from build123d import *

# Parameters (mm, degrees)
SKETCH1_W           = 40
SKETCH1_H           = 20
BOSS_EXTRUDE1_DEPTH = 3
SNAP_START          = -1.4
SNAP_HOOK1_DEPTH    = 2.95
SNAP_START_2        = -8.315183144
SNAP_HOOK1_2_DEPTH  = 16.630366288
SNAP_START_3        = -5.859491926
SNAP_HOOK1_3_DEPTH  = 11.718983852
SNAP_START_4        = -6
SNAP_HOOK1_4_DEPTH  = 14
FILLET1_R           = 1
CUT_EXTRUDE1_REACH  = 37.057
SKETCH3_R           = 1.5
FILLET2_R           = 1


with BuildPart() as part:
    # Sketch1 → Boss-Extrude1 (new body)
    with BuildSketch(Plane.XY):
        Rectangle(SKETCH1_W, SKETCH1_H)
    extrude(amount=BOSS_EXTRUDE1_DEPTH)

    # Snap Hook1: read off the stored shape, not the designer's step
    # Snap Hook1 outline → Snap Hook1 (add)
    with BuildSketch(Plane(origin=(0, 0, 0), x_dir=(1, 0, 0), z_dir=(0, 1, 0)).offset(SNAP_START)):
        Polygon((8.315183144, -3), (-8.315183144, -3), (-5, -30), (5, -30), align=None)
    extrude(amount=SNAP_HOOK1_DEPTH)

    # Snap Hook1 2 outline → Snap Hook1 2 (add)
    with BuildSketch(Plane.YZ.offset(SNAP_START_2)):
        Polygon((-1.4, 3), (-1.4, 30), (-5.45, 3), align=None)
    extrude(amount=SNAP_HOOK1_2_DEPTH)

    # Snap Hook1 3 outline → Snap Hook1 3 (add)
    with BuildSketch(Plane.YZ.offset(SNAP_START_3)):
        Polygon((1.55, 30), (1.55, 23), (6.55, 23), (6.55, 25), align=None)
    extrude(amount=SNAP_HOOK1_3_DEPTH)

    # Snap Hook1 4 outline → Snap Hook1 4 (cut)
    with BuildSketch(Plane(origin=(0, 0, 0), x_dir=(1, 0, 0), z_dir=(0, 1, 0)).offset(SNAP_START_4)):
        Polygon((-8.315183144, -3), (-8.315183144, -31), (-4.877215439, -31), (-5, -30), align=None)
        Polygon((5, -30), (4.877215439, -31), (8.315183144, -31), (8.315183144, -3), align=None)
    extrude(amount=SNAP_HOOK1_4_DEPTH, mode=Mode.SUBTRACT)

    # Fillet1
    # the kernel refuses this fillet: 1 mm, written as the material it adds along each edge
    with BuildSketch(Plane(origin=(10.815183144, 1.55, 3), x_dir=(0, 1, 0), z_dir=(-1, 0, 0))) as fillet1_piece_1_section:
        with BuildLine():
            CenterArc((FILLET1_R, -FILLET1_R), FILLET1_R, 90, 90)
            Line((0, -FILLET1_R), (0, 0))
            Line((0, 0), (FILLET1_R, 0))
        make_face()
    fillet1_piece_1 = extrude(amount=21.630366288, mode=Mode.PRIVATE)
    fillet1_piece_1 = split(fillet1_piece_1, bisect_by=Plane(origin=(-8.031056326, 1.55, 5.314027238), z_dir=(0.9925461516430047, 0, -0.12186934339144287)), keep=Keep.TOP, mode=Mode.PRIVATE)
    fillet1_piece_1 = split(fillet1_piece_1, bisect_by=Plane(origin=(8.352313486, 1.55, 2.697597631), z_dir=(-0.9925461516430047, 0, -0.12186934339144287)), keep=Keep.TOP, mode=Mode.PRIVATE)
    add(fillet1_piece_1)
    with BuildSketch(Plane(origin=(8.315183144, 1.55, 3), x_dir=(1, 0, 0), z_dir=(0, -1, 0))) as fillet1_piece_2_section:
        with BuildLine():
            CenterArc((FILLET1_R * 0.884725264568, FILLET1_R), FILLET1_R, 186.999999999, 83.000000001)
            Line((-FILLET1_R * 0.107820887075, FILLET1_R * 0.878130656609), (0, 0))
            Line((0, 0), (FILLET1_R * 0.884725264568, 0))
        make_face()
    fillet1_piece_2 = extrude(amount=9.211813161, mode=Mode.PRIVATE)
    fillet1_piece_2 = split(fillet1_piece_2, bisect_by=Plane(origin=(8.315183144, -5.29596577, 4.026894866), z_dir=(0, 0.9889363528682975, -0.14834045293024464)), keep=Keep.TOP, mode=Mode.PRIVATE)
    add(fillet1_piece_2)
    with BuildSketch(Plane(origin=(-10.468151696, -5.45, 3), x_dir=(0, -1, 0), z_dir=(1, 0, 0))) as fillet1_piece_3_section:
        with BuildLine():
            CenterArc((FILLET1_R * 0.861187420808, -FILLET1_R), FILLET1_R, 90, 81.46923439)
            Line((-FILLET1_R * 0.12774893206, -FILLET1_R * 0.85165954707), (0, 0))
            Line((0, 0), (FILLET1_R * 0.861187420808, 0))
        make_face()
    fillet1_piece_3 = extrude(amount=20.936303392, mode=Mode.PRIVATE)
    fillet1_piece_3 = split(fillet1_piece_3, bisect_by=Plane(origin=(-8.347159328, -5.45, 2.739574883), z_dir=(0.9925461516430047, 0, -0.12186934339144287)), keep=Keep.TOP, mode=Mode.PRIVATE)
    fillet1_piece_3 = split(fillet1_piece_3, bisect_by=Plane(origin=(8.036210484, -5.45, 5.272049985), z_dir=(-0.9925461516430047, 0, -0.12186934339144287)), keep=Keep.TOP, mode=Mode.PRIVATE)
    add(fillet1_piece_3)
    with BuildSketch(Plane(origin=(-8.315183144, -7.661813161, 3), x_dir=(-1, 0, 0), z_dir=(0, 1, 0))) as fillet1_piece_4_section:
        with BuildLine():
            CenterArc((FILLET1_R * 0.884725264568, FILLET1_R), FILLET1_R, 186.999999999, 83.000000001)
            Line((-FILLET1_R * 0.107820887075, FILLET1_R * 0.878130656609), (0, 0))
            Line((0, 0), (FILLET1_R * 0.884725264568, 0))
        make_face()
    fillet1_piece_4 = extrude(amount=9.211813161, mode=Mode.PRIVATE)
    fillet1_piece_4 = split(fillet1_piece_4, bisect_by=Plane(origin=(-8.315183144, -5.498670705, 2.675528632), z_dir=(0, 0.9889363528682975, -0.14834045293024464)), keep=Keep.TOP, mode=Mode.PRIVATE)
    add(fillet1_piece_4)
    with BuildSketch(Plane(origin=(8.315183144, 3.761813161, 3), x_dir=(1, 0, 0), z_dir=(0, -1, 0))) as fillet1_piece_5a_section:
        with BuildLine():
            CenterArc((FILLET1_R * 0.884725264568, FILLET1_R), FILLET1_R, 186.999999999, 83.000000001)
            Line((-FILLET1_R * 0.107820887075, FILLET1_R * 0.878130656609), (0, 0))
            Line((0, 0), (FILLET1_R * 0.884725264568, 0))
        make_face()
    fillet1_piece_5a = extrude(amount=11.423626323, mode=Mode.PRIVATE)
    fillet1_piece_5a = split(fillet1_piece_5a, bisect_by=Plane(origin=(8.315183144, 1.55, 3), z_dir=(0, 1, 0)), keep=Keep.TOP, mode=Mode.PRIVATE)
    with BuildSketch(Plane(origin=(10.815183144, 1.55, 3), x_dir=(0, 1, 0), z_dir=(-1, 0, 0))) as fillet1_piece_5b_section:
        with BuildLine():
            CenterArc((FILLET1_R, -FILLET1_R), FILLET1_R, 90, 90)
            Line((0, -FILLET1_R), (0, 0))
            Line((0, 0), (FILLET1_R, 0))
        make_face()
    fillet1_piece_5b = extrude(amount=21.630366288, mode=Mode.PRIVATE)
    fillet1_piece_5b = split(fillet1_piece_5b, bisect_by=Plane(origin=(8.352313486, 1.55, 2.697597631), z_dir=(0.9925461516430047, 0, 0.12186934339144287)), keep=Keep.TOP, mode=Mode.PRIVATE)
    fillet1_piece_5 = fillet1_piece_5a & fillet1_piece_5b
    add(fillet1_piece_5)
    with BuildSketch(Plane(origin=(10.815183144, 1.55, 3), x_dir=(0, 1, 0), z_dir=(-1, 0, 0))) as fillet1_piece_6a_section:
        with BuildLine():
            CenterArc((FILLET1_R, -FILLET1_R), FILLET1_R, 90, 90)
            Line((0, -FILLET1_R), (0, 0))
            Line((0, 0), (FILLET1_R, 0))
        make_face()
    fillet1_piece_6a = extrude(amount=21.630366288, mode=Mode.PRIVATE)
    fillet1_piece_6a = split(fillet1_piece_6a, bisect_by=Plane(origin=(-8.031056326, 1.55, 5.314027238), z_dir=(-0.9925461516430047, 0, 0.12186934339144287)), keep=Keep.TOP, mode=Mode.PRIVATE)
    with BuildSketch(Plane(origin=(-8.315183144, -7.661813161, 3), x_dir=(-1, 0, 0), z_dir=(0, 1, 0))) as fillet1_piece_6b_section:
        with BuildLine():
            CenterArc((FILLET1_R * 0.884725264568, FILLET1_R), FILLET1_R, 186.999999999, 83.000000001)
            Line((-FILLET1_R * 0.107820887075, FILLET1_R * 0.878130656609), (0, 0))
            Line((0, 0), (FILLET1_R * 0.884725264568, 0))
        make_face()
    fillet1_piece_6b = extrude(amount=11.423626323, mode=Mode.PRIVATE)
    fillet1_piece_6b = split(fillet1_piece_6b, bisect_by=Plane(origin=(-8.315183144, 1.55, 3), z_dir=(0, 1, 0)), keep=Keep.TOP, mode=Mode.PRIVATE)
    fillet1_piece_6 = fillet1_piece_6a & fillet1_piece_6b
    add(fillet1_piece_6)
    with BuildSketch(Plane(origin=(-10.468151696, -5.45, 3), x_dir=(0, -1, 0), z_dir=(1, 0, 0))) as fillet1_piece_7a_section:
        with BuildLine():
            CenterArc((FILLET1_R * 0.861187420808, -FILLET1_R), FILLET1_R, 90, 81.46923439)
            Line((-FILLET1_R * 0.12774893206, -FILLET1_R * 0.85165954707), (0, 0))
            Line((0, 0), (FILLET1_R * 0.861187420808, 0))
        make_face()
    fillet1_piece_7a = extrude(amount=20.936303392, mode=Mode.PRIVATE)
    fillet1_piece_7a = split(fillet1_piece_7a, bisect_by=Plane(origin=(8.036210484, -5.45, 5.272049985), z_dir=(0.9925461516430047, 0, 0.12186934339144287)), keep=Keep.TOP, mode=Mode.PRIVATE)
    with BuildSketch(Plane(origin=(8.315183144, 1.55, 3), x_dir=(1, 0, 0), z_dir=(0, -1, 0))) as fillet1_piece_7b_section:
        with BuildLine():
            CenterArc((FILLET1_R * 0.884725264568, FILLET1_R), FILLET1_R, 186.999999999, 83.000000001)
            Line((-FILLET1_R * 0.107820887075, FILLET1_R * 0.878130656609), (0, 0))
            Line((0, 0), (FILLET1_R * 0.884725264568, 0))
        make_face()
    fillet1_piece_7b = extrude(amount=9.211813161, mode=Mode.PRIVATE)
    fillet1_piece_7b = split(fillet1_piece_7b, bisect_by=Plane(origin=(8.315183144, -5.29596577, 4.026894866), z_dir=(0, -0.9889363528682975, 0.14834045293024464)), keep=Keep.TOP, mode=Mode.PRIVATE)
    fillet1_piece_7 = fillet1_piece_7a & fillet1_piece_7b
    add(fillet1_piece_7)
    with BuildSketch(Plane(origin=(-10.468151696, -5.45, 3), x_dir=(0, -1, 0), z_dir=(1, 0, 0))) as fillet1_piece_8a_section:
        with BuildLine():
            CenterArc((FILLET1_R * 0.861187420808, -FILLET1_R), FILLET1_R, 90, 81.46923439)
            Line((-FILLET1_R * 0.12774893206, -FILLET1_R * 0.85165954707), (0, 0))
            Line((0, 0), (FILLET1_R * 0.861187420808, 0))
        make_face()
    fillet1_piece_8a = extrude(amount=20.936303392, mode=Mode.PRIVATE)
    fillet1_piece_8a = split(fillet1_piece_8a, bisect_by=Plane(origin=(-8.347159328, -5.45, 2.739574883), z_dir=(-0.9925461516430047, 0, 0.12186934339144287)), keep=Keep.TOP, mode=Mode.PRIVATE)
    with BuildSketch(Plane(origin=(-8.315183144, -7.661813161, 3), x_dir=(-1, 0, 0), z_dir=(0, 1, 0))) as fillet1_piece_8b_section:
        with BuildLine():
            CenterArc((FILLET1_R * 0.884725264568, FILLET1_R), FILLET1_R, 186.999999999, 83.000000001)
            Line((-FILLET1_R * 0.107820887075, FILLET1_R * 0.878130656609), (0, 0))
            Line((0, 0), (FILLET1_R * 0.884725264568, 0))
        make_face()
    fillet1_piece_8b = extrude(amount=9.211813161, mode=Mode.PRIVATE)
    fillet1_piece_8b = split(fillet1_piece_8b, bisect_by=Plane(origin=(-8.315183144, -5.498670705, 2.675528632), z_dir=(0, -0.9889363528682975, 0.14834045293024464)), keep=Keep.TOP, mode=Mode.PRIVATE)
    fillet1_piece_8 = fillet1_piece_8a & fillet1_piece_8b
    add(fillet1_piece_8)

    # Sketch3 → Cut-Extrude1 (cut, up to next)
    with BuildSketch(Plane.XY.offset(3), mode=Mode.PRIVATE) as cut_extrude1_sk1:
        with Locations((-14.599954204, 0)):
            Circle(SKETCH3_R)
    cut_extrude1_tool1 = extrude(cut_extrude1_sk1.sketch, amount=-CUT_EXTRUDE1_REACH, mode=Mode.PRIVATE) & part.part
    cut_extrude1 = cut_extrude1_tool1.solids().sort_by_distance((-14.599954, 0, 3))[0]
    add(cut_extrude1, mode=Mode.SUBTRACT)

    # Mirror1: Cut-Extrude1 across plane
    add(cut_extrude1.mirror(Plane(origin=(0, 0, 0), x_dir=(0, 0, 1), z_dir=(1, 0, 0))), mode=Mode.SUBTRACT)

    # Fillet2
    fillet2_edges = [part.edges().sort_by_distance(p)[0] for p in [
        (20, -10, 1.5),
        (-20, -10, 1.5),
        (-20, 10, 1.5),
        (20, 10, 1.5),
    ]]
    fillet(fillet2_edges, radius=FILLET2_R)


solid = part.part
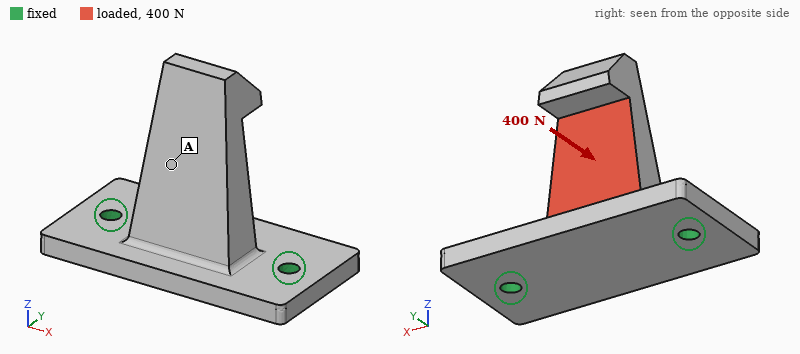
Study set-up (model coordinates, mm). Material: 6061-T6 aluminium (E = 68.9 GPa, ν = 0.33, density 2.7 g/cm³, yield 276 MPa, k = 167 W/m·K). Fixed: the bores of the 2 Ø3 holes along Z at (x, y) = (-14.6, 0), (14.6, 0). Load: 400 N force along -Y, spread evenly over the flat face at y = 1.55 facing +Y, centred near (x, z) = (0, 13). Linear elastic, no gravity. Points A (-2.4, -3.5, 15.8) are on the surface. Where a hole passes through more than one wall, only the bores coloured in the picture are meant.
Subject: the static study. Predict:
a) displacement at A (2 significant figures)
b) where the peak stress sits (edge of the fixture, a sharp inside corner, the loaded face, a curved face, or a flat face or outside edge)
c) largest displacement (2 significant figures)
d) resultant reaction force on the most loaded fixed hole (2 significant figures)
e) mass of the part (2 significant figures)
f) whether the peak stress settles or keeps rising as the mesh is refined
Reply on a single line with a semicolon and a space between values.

0.076 mm; edge of the fixture; 0.16 mm; 200 N; 12 g; keeps rising
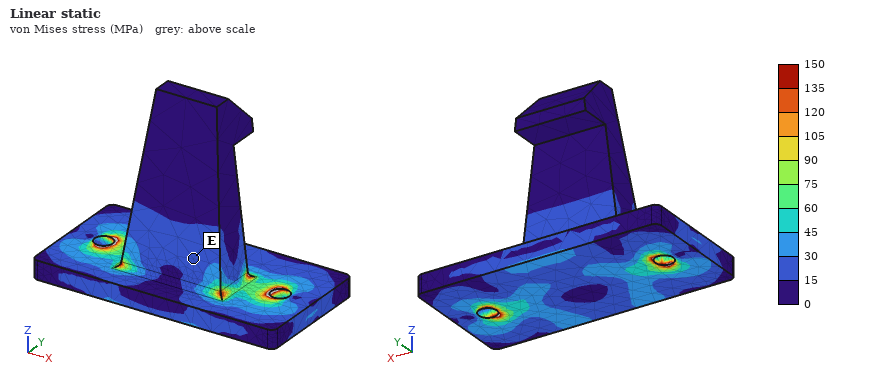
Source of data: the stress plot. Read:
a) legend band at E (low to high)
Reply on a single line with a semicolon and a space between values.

15 to 30 MPa
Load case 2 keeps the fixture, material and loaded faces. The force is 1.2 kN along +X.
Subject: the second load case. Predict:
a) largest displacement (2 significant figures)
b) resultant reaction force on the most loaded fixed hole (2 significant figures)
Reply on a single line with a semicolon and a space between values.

67 µm; 850 N
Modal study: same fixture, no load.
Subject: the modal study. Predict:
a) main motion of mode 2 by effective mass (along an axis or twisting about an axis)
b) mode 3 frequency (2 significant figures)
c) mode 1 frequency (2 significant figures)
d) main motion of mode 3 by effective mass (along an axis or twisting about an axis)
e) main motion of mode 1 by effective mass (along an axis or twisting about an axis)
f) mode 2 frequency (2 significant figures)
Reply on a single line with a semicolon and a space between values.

along X; 13 kHz; 3700 Hz; along Z; along Y; 9700 Hz
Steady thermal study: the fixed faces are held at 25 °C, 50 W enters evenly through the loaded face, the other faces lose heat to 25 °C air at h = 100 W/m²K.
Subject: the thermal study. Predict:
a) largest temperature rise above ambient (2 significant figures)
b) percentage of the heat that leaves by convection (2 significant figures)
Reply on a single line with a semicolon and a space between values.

59 K; 14 %
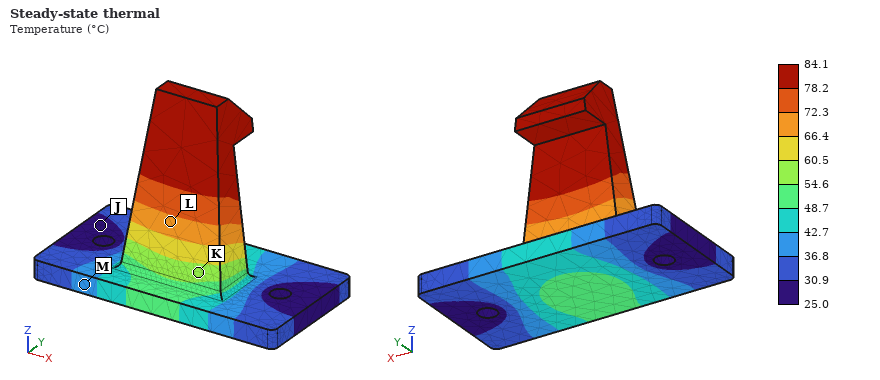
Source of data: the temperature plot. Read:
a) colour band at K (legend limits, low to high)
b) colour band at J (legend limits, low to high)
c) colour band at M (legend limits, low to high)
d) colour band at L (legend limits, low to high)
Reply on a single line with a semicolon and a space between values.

54.6 to 60.5 °C; 25.0 to 30.9 °C; 36.8 to 42.7 °C; 66.4 to 72.3 °C
